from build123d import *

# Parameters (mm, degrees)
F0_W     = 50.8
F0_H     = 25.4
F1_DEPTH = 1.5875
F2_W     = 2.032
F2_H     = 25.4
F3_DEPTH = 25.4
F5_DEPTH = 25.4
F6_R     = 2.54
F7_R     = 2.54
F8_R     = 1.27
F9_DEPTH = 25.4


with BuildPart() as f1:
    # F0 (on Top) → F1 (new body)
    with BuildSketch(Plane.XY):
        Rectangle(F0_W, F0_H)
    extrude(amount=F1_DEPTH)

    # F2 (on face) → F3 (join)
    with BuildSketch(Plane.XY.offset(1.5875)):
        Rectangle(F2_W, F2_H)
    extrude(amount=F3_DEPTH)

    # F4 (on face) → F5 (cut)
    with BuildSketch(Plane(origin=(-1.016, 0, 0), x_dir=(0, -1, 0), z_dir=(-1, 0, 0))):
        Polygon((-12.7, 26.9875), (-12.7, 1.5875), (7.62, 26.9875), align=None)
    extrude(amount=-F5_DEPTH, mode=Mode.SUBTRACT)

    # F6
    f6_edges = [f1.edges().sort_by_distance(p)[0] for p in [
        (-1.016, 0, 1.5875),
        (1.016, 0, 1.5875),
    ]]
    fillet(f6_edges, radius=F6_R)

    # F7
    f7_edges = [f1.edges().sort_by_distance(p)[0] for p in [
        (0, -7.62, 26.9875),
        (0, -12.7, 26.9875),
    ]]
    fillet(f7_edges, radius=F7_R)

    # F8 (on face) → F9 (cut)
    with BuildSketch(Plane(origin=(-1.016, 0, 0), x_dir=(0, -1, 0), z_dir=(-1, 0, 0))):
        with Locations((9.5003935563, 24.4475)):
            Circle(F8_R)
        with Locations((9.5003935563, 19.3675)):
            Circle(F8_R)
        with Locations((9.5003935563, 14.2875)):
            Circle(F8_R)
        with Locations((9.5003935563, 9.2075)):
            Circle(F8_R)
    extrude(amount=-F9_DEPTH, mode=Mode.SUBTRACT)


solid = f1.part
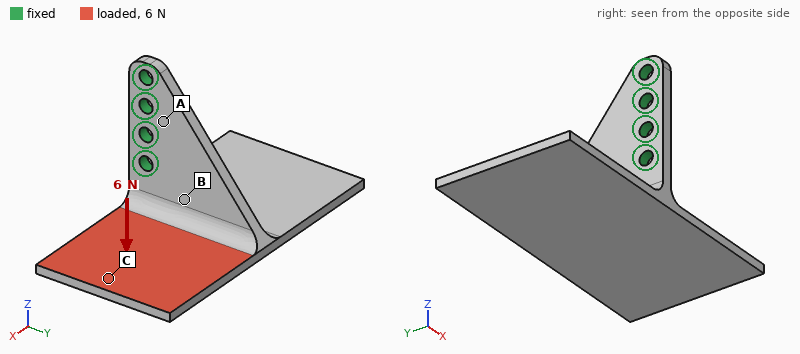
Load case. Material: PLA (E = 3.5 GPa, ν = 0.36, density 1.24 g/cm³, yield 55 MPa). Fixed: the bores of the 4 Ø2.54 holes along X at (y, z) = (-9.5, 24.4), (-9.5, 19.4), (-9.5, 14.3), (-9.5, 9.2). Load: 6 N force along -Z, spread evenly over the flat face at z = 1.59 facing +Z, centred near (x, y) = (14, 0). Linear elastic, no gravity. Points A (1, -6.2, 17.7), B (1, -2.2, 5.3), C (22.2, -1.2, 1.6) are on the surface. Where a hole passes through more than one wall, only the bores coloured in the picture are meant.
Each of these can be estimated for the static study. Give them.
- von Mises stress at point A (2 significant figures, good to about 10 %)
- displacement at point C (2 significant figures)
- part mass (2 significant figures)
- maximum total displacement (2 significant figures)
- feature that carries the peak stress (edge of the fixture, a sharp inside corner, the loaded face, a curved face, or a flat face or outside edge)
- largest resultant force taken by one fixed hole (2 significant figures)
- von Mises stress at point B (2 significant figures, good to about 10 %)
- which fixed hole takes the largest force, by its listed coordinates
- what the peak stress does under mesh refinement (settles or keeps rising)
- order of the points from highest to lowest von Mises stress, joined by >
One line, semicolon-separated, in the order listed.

1.3 MPa; 0.60 mm; 3.5 g; 0.74 mm; edge of the fixture; 7.6 N; 5.6 MPa; (-9.5, 9.2); keeps rising; B > A > C
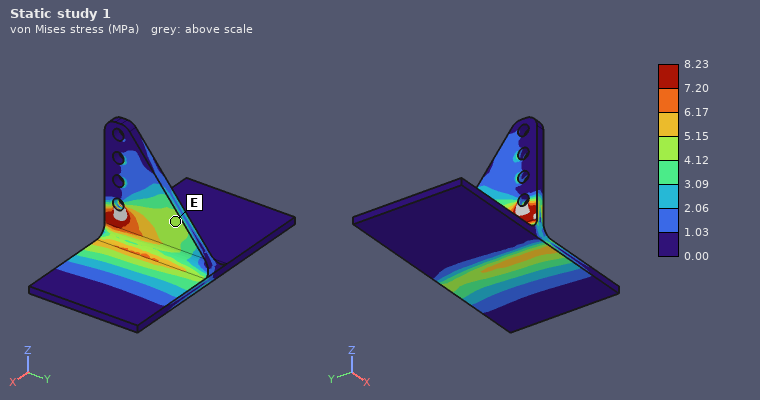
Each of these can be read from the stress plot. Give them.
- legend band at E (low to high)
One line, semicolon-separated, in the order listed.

4.12 to 5.15 MPa
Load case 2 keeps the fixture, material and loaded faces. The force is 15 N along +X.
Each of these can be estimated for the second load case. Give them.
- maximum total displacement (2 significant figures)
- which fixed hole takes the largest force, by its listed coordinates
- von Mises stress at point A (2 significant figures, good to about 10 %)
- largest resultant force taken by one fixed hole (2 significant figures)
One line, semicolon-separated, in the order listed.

0.68 mm; (-9.5, 9.2); 2.7 MPa; 20 N
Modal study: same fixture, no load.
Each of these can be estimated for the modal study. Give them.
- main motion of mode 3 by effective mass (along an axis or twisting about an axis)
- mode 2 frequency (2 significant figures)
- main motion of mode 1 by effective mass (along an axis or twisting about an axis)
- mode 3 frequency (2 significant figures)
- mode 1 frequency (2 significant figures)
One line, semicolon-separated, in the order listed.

along Z; 570 Hz; along X; 800 Hz; 390 Hz
